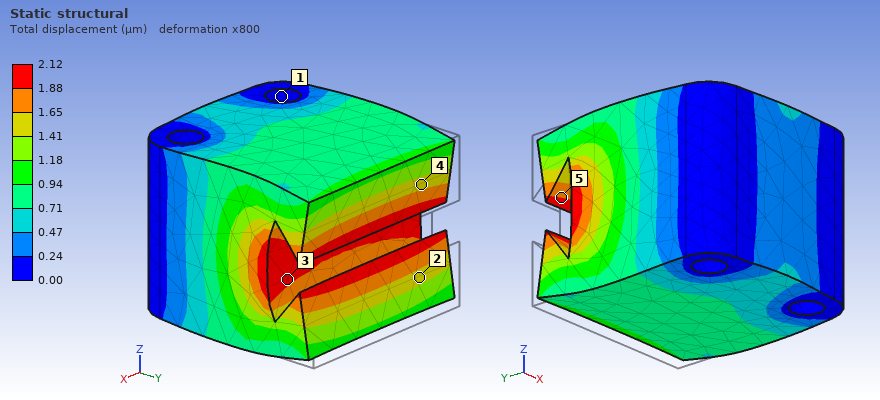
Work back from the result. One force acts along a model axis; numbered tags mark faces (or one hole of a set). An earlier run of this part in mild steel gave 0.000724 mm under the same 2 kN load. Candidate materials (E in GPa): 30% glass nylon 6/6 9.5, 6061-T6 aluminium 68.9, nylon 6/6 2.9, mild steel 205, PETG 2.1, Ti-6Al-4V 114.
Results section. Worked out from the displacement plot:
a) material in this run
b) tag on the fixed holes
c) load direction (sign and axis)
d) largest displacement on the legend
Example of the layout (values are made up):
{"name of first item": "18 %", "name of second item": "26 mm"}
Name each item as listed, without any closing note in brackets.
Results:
{"material in this run": "6061-T6 aluminium", "tag on the fixed holes": "1", "load direction": "-Y", "largest displacement on the legend": "2.12 µm"}
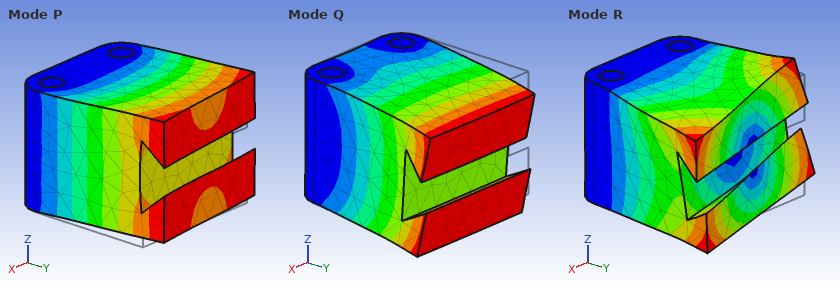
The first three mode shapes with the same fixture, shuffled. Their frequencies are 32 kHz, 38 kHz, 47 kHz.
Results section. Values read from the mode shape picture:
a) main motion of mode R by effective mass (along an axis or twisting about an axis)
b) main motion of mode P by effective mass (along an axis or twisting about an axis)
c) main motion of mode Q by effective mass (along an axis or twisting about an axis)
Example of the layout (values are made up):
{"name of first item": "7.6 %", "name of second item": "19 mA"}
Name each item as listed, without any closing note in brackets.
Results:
{"main motion of mode R by effective mass": "twisting about Y", "main motion of mode P by effective mass": "along X", "main motion of mode Q by effective mass": "along Z"}
